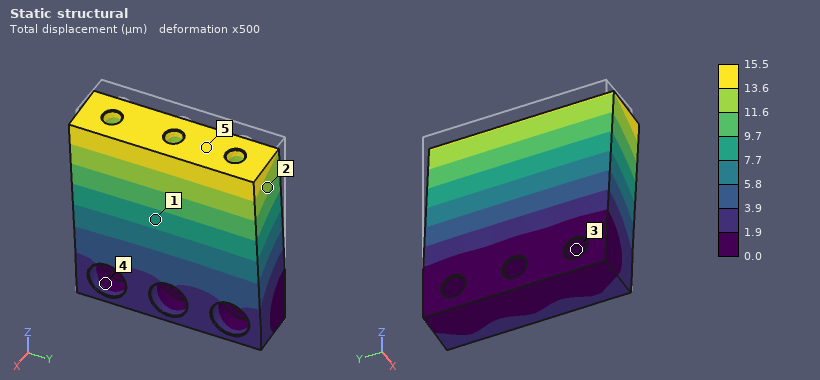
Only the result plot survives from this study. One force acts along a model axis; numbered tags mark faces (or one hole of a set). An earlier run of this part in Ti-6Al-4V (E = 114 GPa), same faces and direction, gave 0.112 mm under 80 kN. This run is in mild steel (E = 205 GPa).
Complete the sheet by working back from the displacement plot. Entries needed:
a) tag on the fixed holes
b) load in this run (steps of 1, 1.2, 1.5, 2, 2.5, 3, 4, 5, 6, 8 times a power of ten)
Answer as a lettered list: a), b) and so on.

a) 3
b) 20 kN
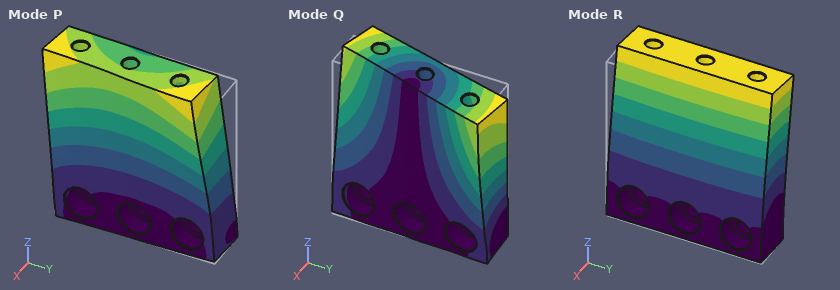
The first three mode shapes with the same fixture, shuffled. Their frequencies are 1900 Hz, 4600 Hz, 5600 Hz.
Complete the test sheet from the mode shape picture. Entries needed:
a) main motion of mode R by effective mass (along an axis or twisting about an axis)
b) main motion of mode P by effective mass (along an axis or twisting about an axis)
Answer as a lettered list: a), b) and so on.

a) along X
b) along Y
